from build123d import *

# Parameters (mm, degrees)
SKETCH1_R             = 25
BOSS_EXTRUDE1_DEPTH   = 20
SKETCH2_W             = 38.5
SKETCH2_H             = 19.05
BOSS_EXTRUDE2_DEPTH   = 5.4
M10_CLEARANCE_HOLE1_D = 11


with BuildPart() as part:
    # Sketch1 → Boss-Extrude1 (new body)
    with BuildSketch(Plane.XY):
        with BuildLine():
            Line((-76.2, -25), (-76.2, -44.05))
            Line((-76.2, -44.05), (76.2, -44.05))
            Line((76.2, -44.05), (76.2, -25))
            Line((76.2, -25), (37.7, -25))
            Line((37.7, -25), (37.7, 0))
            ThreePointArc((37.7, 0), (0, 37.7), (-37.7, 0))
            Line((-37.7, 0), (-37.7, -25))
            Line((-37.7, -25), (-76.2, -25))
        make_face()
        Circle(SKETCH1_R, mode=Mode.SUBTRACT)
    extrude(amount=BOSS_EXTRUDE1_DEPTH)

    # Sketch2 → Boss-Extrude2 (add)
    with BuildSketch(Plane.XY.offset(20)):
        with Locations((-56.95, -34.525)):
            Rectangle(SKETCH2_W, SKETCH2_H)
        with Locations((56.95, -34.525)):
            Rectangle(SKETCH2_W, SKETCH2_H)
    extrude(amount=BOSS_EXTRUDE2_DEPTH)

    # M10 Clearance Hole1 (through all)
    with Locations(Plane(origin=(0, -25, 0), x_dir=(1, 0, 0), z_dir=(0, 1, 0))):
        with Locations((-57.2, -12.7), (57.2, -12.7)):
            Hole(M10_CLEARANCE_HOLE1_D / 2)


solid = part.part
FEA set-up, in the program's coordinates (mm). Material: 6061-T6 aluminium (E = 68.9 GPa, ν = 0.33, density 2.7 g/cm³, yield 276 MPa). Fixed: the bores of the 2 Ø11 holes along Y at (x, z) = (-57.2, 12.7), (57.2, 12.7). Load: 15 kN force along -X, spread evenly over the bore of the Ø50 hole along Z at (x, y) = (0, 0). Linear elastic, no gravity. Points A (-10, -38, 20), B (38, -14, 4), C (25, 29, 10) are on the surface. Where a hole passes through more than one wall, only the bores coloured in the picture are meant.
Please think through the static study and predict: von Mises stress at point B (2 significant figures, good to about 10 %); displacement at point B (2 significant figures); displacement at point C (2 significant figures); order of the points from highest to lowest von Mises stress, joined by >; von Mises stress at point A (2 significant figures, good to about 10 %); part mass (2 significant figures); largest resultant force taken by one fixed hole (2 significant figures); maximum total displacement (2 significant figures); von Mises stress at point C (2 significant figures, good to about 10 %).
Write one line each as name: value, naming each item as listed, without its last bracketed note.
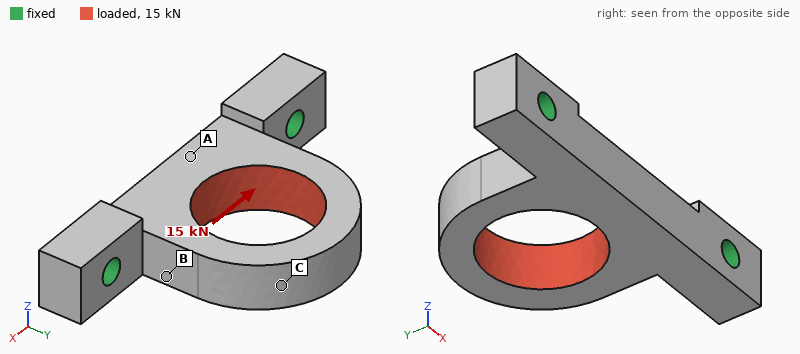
von Mises stress at point B: 76 MPa
displacement at point B: 0.043 mm
displacement at point C: 0.16 mm
order of the points from highest to lowest von Mises stress, joined by >: B > C > A
von Mises stress at point A: 19 MPa
part mass: 280 g
largest resultant force taken by one fixed hole: 9.3 kN
maximum total displacement: 0.17 mm
von Mises stress at point C: 49 MPa
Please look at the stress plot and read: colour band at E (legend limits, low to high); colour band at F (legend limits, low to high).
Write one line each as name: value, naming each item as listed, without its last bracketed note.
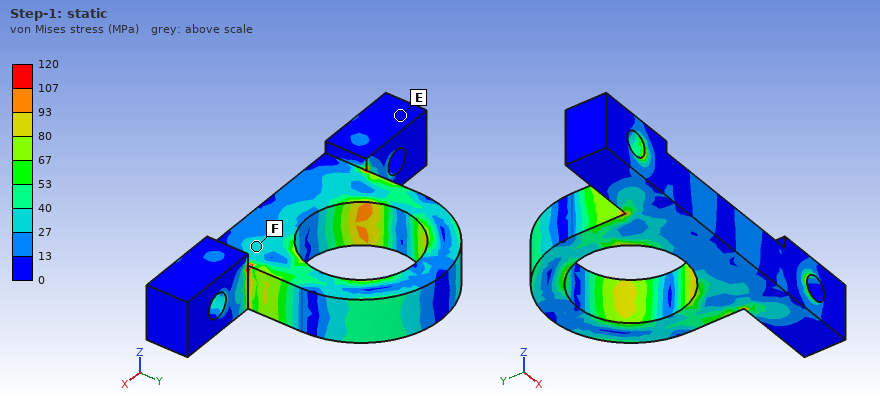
colour band at E: 0 to 13 MPa
colour band at F: 27 to 40 MPa
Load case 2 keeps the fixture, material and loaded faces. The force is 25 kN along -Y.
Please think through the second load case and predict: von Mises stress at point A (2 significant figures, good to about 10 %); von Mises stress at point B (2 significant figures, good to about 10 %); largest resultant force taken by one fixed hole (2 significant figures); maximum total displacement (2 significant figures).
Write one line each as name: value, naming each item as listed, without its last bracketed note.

von Mises stress at point A: 23 MPa
von Mises stress at point B: 74 MPa
largest resultant force taken by one fixed hole: 13 kN
maximum total displacement: 0.10 mm
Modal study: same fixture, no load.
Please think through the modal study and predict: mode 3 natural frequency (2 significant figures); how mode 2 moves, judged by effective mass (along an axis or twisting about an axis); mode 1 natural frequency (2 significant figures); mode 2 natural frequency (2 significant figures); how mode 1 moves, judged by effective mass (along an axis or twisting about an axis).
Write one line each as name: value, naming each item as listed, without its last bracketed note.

mode 3 natural frequency: 5400 Hz
how mode 2 moves, judged by effective mass: along X
mode 1 natural frequency: 2000 Hz
mode 2 natural frequency: 4500 Hz
how mode 1 moves, judged by effective mass: along Z
